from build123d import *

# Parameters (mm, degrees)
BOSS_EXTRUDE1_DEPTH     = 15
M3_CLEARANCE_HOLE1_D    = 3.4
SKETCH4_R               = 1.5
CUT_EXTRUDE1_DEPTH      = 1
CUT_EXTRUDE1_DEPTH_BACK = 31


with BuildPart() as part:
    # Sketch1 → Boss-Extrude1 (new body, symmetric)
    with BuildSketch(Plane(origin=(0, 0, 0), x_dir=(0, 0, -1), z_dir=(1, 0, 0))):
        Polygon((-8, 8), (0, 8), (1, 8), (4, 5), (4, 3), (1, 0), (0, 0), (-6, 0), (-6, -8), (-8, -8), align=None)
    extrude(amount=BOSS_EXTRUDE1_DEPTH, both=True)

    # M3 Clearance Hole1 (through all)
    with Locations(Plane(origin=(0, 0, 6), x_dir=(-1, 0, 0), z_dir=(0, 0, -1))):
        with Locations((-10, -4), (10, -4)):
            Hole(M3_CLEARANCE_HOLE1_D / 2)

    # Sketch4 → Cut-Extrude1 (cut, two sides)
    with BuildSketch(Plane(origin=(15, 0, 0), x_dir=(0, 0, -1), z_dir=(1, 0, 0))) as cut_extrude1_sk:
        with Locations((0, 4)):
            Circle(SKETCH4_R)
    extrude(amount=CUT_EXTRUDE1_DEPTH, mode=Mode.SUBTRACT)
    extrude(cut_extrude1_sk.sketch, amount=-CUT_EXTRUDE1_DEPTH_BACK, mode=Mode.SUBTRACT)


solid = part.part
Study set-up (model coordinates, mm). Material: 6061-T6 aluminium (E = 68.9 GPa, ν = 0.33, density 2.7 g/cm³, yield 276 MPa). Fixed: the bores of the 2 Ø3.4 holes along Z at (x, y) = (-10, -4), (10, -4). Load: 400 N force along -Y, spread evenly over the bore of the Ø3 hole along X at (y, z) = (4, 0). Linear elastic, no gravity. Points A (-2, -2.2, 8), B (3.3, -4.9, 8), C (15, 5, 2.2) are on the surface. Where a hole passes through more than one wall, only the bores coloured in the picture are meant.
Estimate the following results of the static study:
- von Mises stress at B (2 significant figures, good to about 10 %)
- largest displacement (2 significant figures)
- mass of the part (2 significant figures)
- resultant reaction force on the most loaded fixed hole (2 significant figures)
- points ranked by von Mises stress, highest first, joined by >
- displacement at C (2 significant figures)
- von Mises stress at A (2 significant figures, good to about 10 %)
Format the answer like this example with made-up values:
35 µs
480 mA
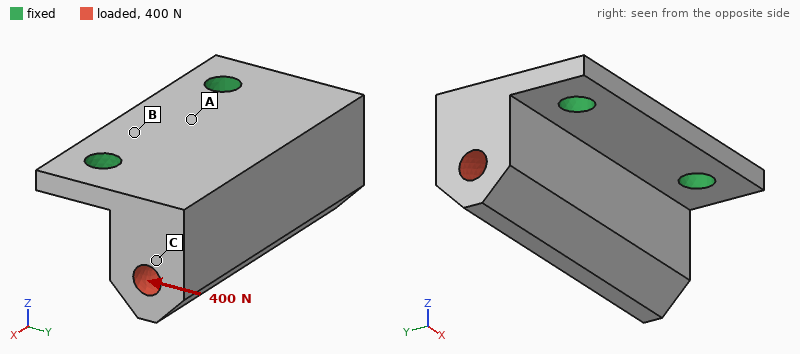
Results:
36 MPa
0.12 mm
7.7 g
200 N
A > B > C
0.072 mm
69 MPa
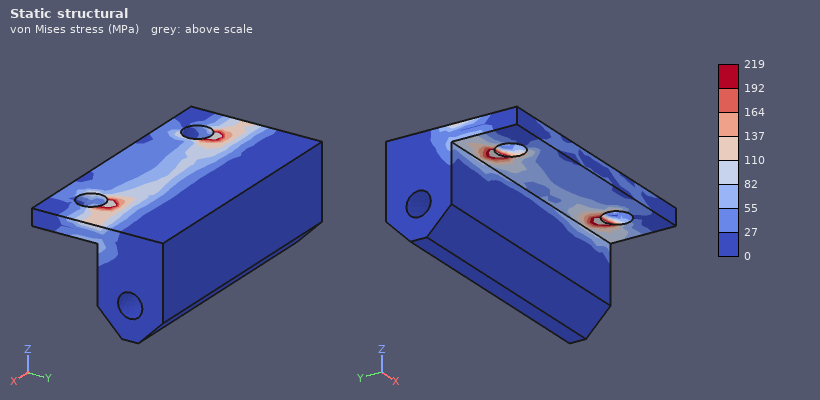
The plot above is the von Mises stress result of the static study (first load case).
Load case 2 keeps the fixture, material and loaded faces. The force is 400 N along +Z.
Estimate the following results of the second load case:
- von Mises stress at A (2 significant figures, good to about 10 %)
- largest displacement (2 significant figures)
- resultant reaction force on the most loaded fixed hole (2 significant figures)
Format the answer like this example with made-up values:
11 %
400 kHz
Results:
47 MPa
89 µm
200 N
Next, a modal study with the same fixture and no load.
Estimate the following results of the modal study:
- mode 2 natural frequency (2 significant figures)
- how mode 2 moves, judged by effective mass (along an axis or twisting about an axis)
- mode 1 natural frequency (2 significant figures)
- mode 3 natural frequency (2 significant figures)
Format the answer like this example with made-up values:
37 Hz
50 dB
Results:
15 kHz
along X
4300 Hz
24 kHz
